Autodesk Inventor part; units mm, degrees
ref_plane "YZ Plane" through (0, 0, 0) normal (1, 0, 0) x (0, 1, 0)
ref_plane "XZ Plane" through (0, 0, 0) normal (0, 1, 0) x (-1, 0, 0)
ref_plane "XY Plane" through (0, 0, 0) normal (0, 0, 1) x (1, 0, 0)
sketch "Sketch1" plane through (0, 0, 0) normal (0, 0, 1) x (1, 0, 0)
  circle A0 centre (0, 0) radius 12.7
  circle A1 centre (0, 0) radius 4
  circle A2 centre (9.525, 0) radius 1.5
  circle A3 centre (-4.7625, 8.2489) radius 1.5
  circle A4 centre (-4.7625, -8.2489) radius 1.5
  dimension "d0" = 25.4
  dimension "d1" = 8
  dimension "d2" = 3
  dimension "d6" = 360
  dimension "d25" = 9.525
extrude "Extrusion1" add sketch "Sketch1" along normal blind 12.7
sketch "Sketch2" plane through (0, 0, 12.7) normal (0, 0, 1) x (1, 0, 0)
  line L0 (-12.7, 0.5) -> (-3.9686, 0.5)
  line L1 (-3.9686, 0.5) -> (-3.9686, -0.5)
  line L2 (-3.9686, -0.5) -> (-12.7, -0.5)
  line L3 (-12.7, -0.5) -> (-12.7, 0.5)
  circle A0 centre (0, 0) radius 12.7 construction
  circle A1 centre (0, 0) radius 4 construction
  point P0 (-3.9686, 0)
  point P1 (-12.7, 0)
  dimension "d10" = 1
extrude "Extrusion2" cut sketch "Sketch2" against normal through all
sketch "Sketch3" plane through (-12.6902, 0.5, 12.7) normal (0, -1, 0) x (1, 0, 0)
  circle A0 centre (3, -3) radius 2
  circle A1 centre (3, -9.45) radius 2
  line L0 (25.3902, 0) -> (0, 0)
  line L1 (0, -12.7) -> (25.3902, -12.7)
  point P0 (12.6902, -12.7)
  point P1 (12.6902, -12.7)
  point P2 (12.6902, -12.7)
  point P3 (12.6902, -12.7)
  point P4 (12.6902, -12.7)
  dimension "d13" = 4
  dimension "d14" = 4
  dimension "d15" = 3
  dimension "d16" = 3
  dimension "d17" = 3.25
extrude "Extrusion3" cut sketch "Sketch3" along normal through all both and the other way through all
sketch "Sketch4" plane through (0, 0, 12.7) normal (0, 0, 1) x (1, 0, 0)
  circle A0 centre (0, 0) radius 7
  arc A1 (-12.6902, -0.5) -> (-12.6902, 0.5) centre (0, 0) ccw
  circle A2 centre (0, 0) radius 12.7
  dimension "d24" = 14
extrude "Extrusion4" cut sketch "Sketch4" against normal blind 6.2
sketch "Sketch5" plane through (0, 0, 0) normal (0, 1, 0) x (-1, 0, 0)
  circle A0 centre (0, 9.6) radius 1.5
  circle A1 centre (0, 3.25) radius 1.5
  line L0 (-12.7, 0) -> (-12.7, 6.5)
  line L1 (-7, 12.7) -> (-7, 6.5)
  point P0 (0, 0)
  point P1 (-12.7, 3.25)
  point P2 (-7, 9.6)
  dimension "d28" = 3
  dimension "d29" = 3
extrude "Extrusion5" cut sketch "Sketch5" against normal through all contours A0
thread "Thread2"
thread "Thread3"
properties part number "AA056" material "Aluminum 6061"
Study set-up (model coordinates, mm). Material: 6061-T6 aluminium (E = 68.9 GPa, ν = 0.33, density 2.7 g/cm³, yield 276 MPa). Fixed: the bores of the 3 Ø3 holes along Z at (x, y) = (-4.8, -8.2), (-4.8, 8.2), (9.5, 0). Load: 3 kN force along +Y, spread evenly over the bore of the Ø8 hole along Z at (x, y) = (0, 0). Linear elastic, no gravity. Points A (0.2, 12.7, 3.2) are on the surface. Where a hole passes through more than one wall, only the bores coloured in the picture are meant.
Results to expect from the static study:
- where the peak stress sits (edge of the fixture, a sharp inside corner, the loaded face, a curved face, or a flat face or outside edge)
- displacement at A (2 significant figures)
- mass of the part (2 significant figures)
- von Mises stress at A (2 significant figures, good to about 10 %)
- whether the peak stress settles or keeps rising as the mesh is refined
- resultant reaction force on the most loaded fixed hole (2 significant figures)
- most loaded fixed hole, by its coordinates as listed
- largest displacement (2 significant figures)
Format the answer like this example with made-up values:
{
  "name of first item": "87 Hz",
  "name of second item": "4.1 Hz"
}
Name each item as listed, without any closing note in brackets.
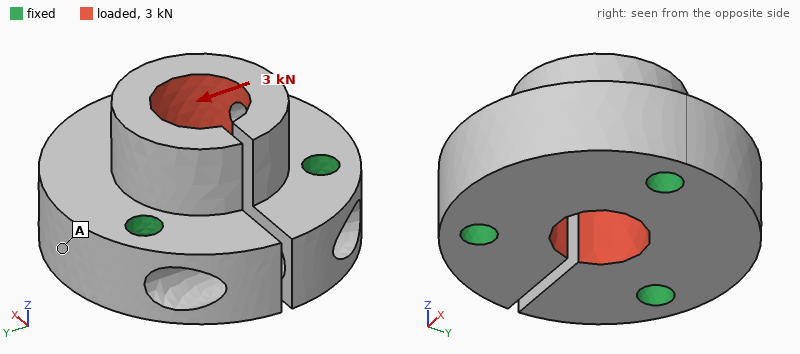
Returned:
{
  "where the peak stress sits": "edge of the fixture",
  "displacement at A": "2.8 µm",
  "mass of the part": "8.6 g",
  "von Mises stress at A": "18 MPa",
  "whether the peak stress settles or keeps rising as the mesh is refined": "keeps rising",
  "resultant reaction force on the most loaded fixed hole": "1.2 kN",
  "most loaded fixed hole, by its coordinates as listed": "(9.5, 0)",
  "largest displacement": "17 µm"
}
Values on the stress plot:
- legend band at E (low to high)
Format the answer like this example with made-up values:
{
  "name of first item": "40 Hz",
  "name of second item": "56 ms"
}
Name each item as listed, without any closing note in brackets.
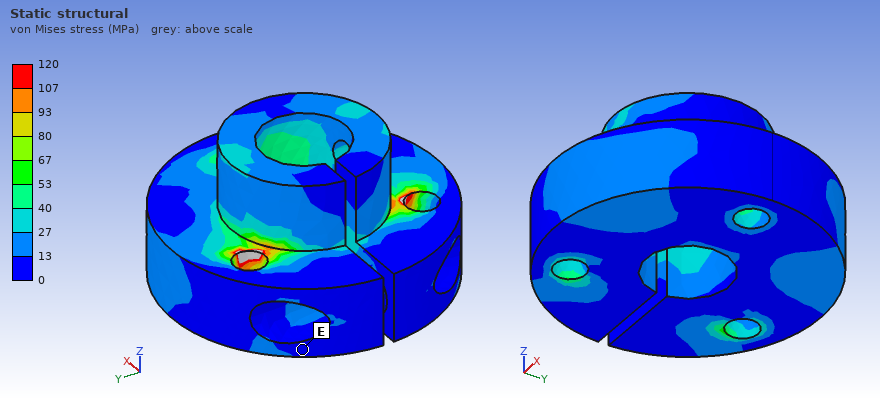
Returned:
{
  "legend band at E": "0 to 13 MPa"
}
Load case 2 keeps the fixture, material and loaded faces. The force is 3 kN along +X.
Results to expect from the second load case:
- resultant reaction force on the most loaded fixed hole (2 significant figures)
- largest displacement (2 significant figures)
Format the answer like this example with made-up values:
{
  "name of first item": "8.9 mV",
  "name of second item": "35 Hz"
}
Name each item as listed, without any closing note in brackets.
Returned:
{
  "resultant reaction force on the most loaded fixed hole": "1.2 kN",
  "largest displacement": "19 µm"
}
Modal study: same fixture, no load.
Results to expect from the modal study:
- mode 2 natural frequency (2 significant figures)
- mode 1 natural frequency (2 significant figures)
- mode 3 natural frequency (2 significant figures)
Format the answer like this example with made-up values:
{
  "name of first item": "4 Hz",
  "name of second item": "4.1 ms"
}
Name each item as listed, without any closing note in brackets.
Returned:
{
  "mode 2 natural frequency": "42 kHz",
  "mode 1 natural frequency": "39 kHz",
  "mode 3 natural frequency": "47 kHz"
}
